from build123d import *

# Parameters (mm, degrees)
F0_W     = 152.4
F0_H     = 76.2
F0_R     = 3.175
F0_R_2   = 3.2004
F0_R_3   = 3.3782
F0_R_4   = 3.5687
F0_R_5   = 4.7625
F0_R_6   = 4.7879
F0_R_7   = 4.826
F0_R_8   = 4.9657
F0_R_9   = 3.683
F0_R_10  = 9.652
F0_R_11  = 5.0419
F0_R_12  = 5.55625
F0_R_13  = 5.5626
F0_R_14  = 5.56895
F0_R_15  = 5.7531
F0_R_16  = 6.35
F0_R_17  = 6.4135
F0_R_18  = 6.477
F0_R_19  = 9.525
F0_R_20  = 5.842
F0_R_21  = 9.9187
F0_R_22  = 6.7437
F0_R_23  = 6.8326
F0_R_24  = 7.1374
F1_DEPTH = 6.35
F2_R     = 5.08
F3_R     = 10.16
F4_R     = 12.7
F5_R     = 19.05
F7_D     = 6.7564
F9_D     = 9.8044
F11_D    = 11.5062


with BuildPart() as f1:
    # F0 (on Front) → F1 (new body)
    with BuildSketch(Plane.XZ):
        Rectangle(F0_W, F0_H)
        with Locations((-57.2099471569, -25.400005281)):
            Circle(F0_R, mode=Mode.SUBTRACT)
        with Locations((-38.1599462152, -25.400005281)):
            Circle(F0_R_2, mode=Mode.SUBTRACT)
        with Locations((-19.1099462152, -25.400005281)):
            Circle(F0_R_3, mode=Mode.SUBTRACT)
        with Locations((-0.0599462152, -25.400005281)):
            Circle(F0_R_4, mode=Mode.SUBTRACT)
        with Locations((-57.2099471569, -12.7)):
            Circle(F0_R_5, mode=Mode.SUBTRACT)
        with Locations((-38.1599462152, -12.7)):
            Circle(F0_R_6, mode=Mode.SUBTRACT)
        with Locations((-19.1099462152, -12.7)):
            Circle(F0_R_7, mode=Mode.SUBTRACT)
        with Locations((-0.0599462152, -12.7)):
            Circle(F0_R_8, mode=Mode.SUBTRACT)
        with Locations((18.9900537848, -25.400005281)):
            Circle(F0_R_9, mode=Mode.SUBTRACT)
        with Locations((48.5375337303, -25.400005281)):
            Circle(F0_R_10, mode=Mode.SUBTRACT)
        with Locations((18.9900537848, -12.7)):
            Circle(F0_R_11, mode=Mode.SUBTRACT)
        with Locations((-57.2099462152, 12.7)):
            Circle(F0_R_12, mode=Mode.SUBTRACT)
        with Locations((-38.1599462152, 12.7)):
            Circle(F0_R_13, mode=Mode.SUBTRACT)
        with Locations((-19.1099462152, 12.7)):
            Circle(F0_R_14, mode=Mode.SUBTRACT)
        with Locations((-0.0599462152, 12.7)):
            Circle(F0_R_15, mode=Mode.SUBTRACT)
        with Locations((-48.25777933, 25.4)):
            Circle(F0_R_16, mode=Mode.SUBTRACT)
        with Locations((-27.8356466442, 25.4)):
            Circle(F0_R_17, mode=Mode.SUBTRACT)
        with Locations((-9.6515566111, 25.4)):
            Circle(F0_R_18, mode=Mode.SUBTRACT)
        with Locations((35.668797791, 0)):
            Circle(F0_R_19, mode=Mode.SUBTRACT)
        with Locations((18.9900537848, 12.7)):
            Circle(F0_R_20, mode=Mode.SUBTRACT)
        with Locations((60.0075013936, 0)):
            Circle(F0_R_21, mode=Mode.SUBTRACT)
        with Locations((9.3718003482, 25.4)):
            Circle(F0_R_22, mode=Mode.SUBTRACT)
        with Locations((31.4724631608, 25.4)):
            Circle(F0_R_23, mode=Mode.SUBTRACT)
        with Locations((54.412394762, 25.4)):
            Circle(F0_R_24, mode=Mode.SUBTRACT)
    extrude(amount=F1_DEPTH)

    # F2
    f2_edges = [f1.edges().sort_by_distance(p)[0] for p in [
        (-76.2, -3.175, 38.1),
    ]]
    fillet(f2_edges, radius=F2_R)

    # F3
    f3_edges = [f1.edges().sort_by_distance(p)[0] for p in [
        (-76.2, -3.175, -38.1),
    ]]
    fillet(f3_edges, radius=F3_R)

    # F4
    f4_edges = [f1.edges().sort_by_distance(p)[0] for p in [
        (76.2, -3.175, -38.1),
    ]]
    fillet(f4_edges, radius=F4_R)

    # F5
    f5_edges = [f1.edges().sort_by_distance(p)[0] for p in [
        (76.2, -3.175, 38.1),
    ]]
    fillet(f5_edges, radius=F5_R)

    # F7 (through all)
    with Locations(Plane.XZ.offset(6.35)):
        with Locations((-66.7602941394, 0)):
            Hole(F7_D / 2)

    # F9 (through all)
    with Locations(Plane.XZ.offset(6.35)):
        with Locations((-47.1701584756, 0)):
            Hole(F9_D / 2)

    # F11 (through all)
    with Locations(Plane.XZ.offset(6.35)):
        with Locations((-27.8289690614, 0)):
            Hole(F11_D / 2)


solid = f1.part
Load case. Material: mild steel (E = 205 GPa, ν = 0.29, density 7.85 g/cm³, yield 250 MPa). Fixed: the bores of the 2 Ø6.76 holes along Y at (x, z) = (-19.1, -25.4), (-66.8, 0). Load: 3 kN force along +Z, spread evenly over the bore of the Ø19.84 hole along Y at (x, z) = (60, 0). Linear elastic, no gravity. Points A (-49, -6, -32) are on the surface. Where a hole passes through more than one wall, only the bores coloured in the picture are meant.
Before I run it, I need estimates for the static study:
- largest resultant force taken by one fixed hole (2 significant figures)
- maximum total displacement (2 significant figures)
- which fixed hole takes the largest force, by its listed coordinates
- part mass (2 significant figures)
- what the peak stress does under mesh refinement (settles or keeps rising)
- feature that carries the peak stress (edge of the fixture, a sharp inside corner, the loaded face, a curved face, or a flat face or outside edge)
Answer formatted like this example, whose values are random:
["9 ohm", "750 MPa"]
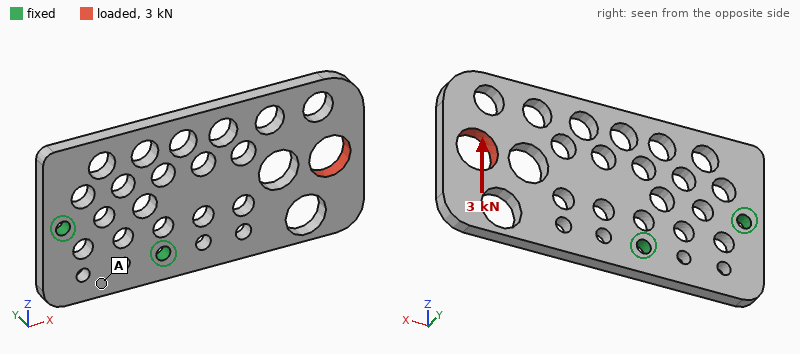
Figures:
["6.3 kN", "88 µm", "(-19.1, -25.4)", "420 g", "keeps rising", "edge of the fixture"]
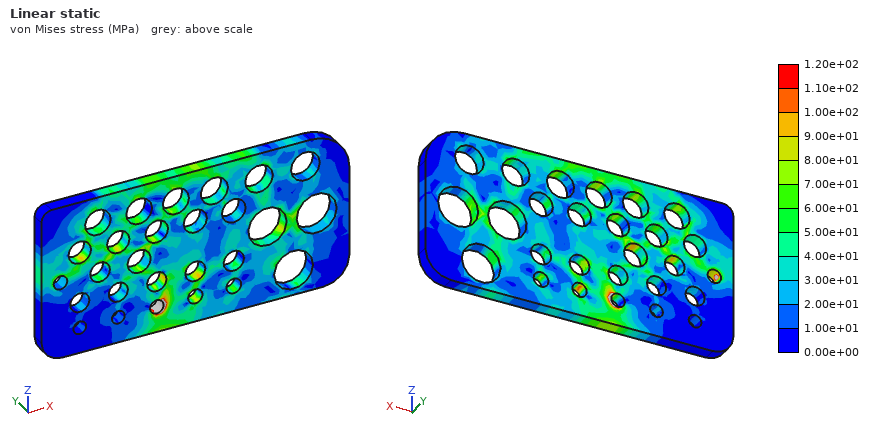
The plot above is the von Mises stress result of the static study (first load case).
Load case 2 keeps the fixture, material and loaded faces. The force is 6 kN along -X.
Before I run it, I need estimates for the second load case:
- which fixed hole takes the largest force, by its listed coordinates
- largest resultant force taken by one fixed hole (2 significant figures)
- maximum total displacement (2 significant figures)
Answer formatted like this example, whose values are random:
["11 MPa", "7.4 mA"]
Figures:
["(-19.1, -25.4)", "3.9 kN", "37 µm"]
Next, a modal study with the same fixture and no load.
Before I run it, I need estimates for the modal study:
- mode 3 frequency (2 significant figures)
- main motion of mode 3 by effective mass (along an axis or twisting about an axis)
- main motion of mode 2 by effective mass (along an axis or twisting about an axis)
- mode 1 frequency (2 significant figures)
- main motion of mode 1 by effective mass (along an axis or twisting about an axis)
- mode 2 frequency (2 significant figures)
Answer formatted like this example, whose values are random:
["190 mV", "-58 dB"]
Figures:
["2100 Hz", "along Y", "twisting about X", "450 Hz", "along Y", "1100 Hz"]
